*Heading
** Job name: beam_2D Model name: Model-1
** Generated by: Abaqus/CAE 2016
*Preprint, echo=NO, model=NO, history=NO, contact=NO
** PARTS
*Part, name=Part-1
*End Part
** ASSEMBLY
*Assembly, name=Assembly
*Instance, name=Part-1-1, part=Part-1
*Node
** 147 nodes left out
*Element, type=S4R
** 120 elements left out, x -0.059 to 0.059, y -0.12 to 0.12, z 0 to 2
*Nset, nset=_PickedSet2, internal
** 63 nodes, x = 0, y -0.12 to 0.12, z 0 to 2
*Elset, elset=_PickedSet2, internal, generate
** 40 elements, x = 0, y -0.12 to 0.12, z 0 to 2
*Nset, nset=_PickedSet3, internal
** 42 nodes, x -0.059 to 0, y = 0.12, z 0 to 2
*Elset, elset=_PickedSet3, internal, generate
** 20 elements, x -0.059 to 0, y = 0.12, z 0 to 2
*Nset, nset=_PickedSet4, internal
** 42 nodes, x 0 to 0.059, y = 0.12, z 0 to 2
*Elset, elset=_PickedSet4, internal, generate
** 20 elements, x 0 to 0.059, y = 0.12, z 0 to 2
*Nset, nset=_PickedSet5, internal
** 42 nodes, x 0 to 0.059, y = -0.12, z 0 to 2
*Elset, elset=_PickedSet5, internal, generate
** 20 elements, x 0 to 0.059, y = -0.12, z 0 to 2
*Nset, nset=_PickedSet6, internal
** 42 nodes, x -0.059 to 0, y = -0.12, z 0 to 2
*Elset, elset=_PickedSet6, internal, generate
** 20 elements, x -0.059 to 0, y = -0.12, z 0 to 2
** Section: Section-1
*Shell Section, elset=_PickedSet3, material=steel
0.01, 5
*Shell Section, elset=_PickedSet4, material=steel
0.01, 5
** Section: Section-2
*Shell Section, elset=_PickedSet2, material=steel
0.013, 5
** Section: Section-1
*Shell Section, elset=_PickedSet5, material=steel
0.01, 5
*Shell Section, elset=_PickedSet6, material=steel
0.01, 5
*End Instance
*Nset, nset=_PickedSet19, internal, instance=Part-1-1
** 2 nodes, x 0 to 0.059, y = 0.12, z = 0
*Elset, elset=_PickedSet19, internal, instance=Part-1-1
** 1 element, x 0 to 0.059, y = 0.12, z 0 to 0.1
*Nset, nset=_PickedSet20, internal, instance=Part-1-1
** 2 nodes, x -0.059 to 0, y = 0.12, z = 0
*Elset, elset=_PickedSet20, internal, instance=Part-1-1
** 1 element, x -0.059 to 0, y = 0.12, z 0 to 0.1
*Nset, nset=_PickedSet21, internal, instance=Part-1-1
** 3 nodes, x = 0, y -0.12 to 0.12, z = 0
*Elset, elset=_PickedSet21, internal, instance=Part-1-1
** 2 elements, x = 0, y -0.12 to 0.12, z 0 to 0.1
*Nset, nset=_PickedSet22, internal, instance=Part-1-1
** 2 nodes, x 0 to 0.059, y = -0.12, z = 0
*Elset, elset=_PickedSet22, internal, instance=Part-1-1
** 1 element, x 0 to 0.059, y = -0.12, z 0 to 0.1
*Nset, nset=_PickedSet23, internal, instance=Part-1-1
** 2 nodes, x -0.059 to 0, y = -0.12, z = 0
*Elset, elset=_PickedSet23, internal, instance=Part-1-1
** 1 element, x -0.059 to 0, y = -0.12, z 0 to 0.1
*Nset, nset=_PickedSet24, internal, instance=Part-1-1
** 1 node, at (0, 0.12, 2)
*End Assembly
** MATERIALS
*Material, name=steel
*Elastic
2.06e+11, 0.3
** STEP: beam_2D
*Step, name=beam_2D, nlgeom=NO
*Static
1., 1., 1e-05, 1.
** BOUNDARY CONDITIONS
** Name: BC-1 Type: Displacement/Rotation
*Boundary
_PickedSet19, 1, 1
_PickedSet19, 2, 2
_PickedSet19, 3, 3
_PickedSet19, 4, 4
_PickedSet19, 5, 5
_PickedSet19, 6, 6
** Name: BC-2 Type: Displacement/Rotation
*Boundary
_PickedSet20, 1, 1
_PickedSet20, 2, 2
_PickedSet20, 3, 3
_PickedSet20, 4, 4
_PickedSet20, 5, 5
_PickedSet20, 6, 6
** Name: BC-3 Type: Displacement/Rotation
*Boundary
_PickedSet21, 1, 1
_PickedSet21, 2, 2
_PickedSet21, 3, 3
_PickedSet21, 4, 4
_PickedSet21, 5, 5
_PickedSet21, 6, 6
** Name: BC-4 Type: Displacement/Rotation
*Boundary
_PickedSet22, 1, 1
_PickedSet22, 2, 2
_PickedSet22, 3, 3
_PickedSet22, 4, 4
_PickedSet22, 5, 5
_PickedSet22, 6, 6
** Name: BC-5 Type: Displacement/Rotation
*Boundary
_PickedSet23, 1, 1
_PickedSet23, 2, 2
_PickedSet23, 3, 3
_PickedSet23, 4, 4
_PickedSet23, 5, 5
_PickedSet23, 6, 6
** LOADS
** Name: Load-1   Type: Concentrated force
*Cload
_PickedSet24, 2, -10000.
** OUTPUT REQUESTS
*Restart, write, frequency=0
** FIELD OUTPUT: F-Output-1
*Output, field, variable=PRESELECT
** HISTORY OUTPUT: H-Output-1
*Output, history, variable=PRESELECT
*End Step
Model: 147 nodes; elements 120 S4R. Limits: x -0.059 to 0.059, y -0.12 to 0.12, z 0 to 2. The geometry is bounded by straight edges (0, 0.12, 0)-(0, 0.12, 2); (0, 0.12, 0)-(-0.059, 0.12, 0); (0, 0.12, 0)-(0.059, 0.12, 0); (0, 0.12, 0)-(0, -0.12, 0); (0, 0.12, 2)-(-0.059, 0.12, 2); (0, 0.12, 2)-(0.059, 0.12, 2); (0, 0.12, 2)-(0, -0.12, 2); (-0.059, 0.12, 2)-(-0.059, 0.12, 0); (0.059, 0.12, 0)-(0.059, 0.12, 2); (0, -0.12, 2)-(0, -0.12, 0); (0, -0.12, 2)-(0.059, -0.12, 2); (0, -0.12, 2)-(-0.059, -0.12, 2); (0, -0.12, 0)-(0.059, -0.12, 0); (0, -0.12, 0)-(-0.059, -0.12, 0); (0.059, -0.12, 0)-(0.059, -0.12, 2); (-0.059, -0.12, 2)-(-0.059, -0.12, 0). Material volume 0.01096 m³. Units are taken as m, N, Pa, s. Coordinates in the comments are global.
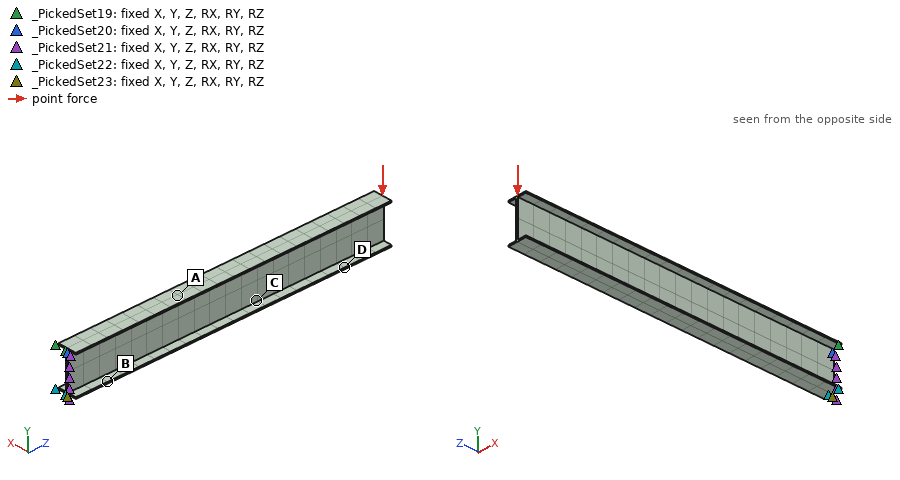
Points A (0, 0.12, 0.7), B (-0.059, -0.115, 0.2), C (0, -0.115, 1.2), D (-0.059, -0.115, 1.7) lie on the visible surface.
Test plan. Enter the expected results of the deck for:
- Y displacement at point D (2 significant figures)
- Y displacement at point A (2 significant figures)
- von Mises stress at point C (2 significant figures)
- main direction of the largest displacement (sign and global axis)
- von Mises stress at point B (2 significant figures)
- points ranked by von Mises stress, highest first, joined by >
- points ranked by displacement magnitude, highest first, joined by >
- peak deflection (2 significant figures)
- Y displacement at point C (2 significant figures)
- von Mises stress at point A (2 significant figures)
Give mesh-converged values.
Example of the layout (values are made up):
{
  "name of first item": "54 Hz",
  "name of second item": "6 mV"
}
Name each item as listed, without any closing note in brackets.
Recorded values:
{
  "Y displacement at point D": "-0.0021 m",
  "Y displacement at point A": "-4.6e-04 m",
  "von Mises stress at point C": "1.9e+07 Pa",
  "main direction of the largest displacement": "-Y",
  "von Mises stress at point B": "4.2e+07 Pa",
  "points ranked by von Mises stress, highest first, joined by >": "B > A > C > D",
  "points ranked by displacement magnitude, highest first, joined by >": "D > C > A > B",
  "peak deflection": "0.0027 m",
  "Y displacement at point C": "-0.0012 m",
  "von Mises stress at point A": "3.2e+07 Pa"
}
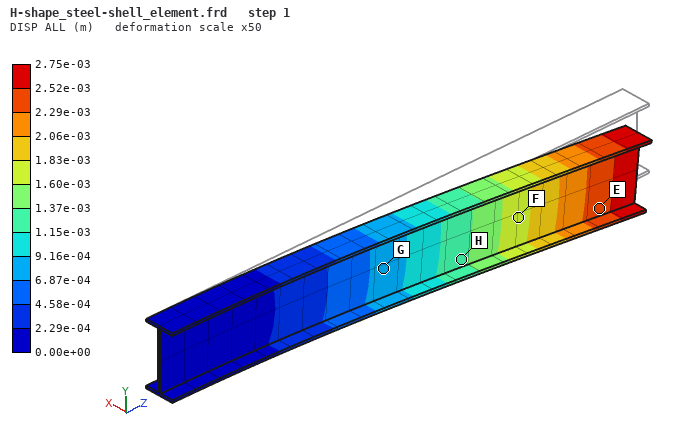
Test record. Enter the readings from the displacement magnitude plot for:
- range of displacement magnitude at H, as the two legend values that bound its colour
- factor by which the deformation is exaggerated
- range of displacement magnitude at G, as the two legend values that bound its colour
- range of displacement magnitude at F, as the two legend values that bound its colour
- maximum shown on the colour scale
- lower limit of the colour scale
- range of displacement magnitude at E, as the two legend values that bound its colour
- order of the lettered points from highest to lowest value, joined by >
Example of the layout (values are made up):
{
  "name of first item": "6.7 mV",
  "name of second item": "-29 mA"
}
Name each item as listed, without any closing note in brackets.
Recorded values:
{
  "range of displacement magnitude at H, as the two legend values that bound its colour": "1.15e-03 to 1.37e-03 m",
  "factor by which the deformation is exaggerated": "50",
  "range of displacement magnitude at G, as the two legend values that bound its colour": "6.87e-04 to 9.16e-04 m",
  "range of displacement magnitude at F, as the two legend values that bound its colour": "1.60e-03 to 1.83e-03 m",
  "maximum shown on the colour scale": "2.75e-03 m",
  "lower limit of the colour scale": "0.00e+00 m",
  "range of displacement magnitude at E, as the two legend values that bound its colour": "2.29e-03 to 2.52e-03 m",
  "order of the lettered points from highest to lowest value, joined by >": "E > F > H > G"
}
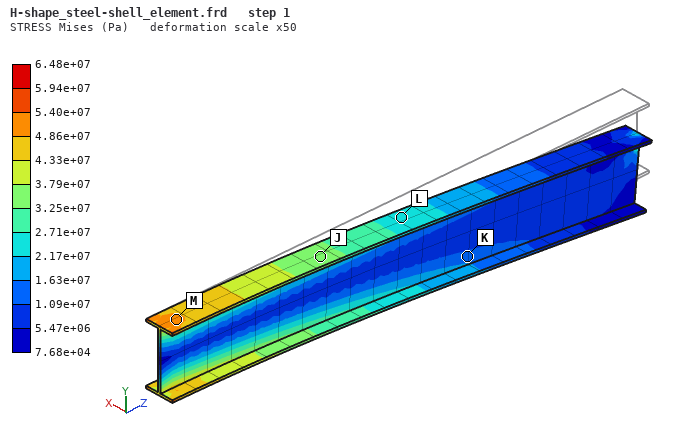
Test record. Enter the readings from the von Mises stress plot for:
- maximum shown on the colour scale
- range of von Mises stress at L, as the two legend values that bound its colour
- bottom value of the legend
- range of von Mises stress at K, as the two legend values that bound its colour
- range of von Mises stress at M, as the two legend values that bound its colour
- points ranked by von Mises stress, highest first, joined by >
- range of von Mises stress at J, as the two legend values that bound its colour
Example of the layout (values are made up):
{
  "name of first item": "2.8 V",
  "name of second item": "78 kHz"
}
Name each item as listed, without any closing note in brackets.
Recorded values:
{
  "maximum shown on the colour scale": "6.48e+07 Pa",
  "range of von Mises stress at L, as the two legend values that bound its colour": "2.17e+07 to 2.71e+07 Pa",
  "bottom value of the legend": "7.68e+04 Pa",
  "range of von Mises stress at K, as the two legend values that bound its colour": "1.09e+07 to 1.63e+07 Pa",
  "range of von Mises stress at M, as the two legend values that bound its colour": "4.86e+07 to 5.40e+07 Pa",
  "points ranked by von Mises stress, highest first, joined by >": "M > J > L > K",
  "range of von Mises stress at J, as the two legend values that bound its colour": "3.25e+07 to 3.79e+07 Pa"
}
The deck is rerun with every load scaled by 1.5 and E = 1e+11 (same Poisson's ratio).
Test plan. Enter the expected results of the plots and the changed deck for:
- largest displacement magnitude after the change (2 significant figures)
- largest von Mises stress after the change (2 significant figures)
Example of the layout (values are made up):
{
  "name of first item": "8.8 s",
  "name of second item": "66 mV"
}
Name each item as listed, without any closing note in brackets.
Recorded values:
{
  "largest displacement magnitude after the change": "0.0085 m",
  "largest von Mises stress after the change": "9.7e+07 Pa"
}
